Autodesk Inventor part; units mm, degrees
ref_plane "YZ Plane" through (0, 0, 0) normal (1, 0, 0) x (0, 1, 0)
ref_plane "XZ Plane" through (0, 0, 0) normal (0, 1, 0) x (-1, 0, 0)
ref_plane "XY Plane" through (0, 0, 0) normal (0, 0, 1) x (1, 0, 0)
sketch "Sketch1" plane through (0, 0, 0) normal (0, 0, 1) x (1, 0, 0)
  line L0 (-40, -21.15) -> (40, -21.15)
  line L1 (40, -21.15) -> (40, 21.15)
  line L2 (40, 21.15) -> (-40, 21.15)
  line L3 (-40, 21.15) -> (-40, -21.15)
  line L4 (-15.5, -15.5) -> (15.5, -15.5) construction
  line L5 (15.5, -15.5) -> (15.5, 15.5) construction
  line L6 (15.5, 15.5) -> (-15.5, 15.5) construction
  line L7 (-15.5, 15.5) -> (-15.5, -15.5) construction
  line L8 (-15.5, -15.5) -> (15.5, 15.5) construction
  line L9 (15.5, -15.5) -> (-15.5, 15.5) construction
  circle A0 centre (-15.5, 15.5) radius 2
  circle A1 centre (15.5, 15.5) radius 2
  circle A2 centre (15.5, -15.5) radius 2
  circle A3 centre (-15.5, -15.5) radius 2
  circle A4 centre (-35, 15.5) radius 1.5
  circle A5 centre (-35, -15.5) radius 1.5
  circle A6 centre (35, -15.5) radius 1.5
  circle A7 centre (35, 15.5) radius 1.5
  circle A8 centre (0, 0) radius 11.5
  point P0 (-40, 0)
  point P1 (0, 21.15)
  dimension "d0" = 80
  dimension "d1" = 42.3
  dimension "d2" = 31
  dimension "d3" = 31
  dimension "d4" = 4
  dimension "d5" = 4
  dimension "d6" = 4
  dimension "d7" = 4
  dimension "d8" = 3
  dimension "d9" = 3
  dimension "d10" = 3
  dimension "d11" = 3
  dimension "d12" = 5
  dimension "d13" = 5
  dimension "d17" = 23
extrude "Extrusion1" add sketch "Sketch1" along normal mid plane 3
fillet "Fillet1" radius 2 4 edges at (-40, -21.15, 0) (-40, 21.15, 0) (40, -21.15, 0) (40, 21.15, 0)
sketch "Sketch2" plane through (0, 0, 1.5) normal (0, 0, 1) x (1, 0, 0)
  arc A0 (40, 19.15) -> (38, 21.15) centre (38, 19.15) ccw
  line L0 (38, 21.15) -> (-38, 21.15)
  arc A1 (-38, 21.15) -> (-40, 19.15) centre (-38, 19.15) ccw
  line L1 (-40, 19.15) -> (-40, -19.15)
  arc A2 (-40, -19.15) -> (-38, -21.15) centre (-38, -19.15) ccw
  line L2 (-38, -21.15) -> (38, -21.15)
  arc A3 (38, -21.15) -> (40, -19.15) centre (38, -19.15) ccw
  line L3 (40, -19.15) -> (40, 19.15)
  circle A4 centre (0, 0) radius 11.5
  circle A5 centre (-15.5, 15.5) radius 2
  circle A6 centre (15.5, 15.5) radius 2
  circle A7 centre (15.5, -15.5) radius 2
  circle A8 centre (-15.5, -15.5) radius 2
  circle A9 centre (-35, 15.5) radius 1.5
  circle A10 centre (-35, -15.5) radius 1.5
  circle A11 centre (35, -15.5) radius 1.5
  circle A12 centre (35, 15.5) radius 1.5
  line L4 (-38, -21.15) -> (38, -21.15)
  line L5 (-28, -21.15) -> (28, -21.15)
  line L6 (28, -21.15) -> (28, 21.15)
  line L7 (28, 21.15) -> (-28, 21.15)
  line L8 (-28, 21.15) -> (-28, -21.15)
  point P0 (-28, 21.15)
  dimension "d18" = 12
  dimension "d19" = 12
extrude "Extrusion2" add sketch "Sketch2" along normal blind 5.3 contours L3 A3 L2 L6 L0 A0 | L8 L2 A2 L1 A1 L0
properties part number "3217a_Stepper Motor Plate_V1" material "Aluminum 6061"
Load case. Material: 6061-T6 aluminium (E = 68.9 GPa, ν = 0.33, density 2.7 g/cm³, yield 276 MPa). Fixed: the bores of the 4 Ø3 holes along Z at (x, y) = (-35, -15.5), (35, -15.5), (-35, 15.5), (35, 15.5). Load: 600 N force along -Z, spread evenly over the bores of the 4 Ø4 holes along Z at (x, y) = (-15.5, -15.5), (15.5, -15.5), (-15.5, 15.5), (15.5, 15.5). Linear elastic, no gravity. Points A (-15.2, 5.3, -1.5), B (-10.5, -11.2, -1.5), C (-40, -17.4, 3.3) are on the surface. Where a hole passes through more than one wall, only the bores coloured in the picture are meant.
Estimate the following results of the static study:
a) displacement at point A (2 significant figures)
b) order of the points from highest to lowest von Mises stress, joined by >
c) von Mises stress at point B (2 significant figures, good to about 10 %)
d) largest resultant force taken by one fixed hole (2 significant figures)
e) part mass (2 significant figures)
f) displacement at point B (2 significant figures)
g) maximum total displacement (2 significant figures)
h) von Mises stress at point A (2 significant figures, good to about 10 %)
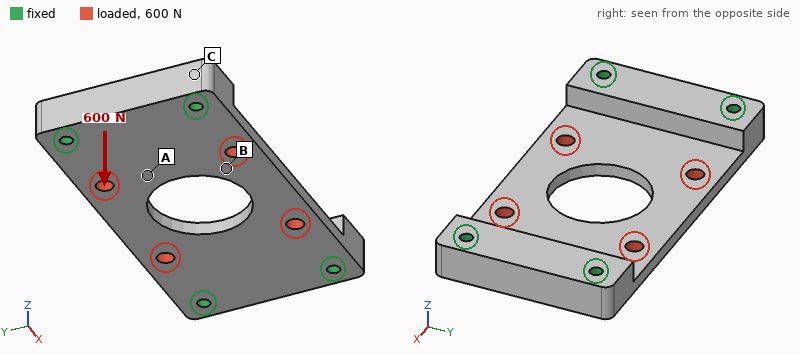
32 µm
B > A > C
18 MPa
170 N
37 g
48 µm
70 µm
11 MPa
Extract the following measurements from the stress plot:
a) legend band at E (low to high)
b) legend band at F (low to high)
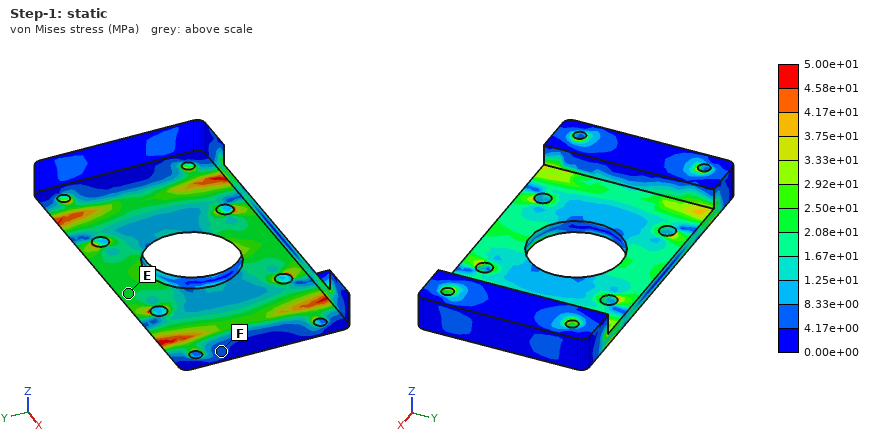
2.08e+01 to 2.50e+01 MPa
4.17e+00 to 8.33e+00 MPa
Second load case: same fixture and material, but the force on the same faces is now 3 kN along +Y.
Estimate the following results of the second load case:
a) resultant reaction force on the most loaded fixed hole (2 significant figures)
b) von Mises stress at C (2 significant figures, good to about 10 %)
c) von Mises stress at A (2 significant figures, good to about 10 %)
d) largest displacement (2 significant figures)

980 N
6.6 MPa
15 MPa
13 µm
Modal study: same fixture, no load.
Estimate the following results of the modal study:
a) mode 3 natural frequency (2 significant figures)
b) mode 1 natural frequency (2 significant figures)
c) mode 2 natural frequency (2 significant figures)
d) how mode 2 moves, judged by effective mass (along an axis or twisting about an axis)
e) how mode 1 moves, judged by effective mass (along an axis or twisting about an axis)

10 kHz
4800 Hz
5700 Hz
twisting about X
along Z
